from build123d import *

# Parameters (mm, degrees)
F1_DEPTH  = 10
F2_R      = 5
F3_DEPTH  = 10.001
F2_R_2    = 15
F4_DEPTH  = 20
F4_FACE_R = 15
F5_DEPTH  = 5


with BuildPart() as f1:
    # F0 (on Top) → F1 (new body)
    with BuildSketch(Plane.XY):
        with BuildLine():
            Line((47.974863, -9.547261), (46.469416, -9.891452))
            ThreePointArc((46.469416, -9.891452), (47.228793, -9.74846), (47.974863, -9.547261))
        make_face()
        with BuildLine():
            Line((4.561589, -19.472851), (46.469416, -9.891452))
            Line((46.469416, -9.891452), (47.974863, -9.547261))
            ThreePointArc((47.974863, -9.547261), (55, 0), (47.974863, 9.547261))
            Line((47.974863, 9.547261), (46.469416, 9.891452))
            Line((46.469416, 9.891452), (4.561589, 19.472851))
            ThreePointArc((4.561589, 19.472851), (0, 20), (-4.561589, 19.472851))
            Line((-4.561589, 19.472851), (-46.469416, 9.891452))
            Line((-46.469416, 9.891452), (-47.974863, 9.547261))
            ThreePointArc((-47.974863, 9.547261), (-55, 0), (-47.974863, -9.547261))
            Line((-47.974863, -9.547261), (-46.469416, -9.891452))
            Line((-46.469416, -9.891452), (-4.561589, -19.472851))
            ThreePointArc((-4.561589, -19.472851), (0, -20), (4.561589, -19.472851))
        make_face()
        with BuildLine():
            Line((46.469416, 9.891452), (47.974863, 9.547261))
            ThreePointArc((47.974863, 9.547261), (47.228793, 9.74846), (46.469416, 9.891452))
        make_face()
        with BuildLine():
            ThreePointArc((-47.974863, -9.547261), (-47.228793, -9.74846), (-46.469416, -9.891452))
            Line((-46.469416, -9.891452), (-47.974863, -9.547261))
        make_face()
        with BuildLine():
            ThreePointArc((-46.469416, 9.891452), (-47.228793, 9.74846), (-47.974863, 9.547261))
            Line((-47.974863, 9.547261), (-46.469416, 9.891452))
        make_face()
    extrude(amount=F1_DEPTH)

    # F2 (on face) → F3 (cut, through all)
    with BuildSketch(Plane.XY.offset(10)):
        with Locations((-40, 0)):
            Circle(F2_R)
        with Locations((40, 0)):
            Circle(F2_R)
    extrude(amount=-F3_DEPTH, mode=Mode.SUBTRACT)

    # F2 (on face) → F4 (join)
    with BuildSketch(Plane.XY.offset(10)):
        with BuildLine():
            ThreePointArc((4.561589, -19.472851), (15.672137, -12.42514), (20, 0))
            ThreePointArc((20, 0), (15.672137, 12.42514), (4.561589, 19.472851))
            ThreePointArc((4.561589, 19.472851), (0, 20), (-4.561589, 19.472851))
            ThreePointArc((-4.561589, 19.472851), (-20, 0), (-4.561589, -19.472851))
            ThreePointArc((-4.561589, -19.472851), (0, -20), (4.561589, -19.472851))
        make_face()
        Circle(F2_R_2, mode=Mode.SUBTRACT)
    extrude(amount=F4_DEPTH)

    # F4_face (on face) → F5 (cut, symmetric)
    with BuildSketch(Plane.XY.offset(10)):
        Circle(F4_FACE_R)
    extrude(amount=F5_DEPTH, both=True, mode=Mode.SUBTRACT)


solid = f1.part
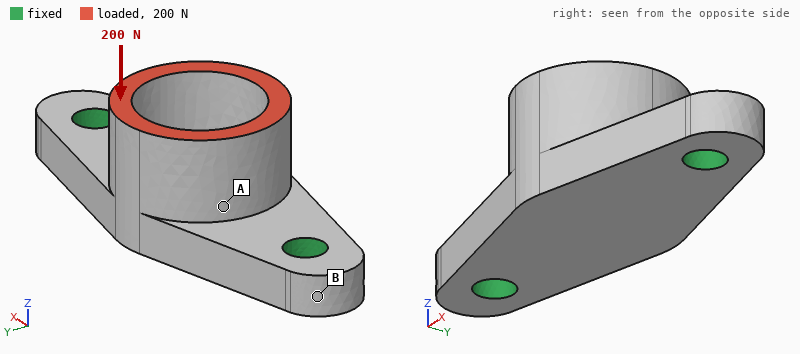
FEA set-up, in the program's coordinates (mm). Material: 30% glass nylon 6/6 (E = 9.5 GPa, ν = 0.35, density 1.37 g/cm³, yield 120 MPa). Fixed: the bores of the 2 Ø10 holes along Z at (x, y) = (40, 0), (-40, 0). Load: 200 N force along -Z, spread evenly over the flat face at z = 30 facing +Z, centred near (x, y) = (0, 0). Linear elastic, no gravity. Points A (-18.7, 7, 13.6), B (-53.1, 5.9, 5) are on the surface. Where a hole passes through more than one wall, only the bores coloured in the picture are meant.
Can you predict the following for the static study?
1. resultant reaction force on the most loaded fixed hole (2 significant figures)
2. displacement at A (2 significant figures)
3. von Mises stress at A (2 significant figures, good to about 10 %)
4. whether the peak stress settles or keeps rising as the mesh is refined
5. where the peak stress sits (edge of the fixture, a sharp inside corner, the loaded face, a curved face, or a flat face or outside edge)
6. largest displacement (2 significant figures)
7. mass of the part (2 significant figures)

100 N
9.6 µm
1.4 MPa
keeps rising
edge of the fixture
16 µm
50 g
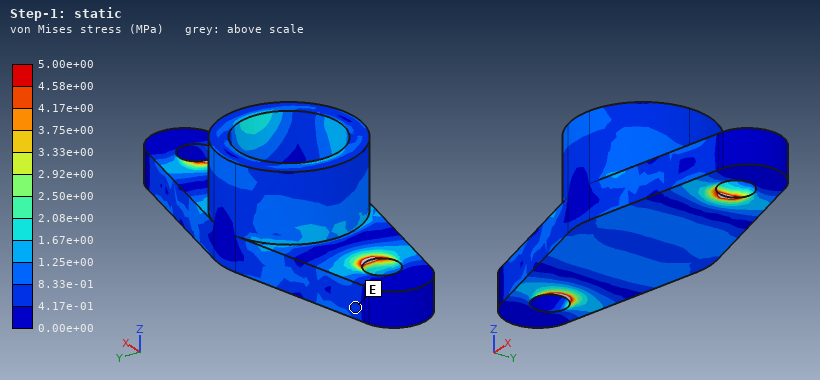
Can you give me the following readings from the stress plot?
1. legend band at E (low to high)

4.17e-01 to 8.33e-01 MPa
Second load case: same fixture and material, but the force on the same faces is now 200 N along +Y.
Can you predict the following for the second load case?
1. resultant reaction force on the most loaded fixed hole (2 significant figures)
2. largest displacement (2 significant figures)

100 N
72 µm
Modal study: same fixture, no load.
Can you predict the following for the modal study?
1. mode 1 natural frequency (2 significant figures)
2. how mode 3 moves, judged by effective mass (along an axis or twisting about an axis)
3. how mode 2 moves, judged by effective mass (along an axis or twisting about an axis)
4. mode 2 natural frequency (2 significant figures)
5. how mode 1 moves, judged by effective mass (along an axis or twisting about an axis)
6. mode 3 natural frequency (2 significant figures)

2700 Hz
along X
along Z
3600 Hz
along Y
6400 Hz
